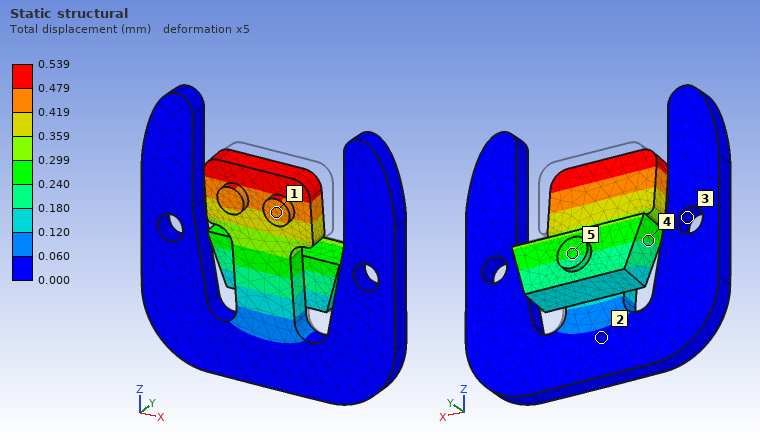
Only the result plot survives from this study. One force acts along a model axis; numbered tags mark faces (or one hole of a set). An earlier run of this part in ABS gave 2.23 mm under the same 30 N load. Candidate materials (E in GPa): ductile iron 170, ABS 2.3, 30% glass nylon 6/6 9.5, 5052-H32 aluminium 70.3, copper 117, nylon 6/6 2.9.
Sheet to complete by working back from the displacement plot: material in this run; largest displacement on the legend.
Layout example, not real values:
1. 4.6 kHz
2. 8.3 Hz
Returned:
1. 30% glass nylon 6/6
2. 0.539 mm
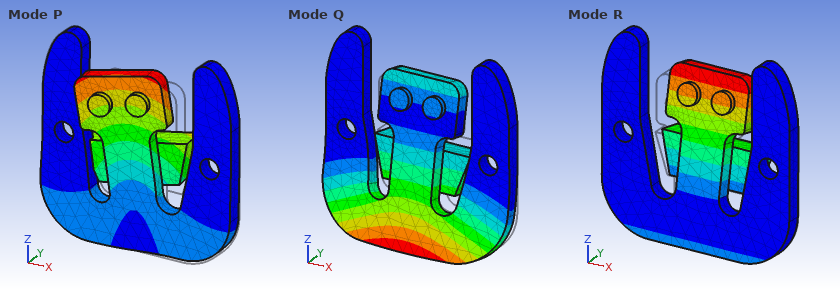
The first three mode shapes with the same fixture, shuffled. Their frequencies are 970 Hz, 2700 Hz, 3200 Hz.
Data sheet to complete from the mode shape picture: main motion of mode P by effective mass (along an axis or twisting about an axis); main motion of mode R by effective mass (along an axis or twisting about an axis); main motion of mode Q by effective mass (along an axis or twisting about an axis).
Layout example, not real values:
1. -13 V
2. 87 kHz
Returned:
1. along X
2. along Y
3. along Y
